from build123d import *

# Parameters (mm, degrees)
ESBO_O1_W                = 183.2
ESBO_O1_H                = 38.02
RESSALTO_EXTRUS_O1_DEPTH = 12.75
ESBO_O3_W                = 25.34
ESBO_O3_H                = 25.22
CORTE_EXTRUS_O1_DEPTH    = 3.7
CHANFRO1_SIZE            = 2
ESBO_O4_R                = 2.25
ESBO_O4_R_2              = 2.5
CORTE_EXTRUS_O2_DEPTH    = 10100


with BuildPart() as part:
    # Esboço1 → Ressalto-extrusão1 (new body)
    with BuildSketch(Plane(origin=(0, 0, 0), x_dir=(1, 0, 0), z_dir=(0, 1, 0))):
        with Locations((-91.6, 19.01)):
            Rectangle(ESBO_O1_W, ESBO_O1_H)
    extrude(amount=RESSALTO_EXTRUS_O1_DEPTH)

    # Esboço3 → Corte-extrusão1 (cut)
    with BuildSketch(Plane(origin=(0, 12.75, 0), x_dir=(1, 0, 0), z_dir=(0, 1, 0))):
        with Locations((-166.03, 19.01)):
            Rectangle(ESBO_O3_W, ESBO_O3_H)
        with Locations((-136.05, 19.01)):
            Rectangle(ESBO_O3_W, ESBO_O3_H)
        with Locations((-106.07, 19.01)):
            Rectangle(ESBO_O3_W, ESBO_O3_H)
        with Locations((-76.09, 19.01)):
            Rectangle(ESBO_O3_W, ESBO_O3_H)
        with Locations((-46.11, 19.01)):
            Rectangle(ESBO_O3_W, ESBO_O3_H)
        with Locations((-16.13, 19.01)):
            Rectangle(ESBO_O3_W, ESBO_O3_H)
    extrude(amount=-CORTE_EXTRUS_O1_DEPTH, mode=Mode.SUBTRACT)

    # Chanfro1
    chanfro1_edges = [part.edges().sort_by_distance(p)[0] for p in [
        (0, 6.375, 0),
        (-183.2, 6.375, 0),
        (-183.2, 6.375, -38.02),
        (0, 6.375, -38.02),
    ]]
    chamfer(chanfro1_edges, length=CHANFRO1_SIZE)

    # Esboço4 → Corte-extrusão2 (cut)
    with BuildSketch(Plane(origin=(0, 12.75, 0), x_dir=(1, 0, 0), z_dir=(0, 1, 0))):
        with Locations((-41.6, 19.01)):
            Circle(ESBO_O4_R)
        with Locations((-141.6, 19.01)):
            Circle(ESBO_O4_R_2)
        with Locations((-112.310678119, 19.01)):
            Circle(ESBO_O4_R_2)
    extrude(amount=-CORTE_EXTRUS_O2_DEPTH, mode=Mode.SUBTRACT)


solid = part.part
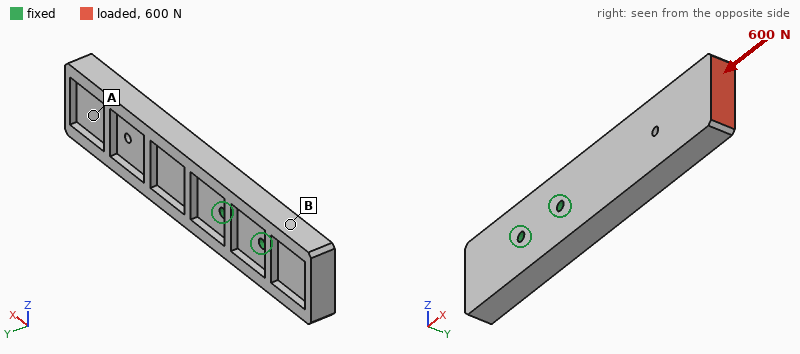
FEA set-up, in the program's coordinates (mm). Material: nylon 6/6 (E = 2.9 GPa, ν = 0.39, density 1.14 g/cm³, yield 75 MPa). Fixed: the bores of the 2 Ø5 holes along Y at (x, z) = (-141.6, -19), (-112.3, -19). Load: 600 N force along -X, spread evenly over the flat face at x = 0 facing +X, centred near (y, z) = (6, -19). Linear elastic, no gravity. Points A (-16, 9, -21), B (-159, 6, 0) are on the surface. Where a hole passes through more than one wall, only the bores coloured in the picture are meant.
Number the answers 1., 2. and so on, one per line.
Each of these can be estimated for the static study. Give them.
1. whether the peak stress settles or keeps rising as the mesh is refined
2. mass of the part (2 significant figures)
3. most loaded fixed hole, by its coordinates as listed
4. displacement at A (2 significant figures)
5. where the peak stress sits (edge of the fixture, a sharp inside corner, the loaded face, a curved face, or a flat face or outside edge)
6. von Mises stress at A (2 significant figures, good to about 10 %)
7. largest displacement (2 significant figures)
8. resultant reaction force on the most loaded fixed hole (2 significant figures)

1. keeps rising
2. 84 g
3. (-112.3, -19)
4. 0.30 mm
5. edge of the fixture
6. 2.7 MPa
7. 0.42 mm
8. 430 N
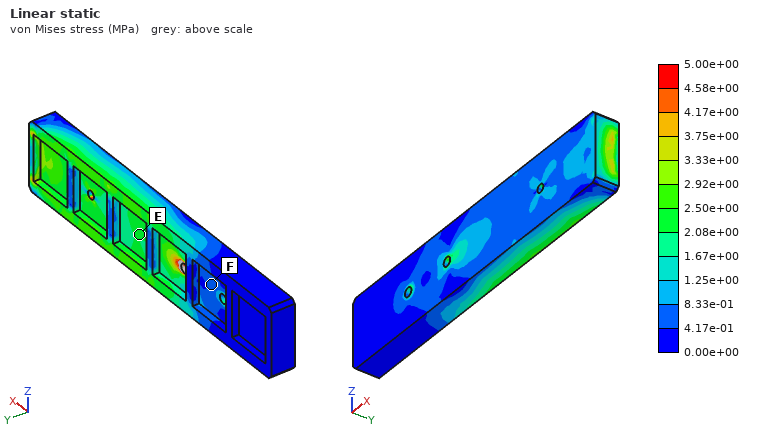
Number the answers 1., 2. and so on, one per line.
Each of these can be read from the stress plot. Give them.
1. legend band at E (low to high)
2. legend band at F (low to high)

1. 2.08e+00 to 2.50e+00 MPa
2. 4.17e-01 to 8.33e-01 MPa
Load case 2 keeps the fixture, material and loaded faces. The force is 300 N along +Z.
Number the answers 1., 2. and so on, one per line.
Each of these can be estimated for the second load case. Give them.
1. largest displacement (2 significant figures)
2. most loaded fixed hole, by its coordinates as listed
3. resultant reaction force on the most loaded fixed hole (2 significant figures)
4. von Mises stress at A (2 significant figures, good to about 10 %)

1. 1.7 mm
2. (-112.3, -19)
3. 1.3 kN
4. 3.6 MPa
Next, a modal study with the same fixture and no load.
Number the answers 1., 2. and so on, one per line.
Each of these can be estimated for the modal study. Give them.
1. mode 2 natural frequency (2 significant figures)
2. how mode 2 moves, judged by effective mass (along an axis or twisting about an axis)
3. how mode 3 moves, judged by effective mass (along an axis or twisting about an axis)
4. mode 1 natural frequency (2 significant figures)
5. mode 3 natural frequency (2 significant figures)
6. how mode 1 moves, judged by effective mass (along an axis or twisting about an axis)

1. 550 Hz
2. along Z
3. twisting about X
4. 210 Hz
5. 860 Hz
6. along Y
